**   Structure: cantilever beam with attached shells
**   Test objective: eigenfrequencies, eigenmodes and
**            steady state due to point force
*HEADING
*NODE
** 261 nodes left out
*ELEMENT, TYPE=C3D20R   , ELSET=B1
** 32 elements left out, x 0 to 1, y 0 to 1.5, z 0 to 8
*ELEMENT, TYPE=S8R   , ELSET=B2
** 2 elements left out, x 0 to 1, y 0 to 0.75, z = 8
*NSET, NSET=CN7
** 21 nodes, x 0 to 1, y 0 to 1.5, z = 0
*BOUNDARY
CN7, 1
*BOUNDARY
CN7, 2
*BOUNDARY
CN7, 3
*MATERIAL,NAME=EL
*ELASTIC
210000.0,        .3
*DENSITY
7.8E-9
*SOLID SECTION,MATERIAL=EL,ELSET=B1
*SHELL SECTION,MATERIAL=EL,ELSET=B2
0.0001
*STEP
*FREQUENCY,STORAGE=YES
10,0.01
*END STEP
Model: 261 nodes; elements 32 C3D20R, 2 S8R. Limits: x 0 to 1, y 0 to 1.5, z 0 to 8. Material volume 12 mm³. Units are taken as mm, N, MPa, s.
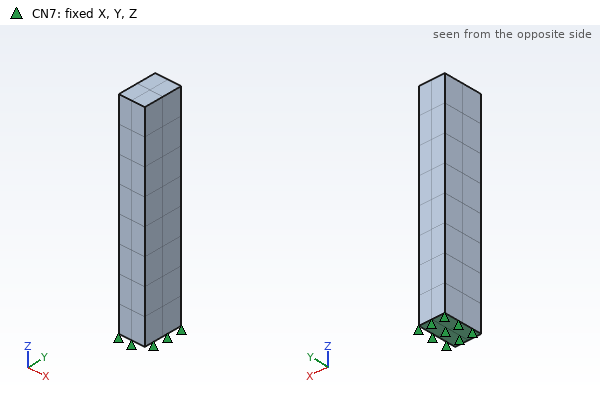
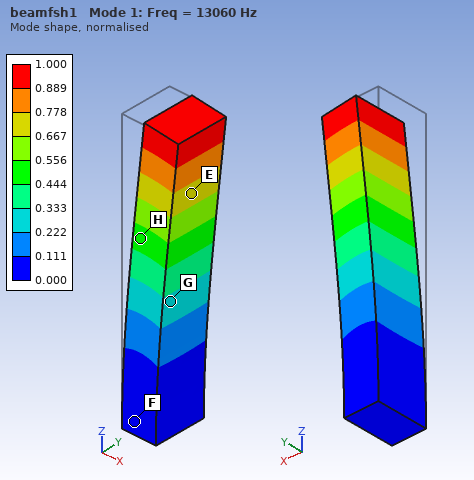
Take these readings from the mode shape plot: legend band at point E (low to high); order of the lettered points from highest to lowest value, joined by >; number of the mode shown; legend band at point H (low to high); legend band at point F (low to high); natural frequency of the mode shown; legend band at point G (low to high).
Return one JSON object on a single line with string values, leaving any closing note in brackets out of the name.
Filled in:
{"legend band at point E": "0.667 to 0.778", "order of the lettered points from highest to lowest value, joined by >": "E > H > G > F", "number of the mode shown": "1", "legend band at point H": "0.444 to 0.556", "legend band at point F": "0.000 to 0.111", "natural frequency of the mode shown": "13060 Hz", "legend band at point G": "0.222 to 0.333"}
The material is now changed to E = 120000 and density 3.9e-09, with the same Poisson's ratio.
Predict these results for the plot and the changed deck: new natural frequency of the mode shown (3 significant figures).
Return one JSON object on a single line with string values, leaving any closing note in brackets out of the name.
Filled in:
{"new natural frequency of the mode shown": "14000 Hz"}
